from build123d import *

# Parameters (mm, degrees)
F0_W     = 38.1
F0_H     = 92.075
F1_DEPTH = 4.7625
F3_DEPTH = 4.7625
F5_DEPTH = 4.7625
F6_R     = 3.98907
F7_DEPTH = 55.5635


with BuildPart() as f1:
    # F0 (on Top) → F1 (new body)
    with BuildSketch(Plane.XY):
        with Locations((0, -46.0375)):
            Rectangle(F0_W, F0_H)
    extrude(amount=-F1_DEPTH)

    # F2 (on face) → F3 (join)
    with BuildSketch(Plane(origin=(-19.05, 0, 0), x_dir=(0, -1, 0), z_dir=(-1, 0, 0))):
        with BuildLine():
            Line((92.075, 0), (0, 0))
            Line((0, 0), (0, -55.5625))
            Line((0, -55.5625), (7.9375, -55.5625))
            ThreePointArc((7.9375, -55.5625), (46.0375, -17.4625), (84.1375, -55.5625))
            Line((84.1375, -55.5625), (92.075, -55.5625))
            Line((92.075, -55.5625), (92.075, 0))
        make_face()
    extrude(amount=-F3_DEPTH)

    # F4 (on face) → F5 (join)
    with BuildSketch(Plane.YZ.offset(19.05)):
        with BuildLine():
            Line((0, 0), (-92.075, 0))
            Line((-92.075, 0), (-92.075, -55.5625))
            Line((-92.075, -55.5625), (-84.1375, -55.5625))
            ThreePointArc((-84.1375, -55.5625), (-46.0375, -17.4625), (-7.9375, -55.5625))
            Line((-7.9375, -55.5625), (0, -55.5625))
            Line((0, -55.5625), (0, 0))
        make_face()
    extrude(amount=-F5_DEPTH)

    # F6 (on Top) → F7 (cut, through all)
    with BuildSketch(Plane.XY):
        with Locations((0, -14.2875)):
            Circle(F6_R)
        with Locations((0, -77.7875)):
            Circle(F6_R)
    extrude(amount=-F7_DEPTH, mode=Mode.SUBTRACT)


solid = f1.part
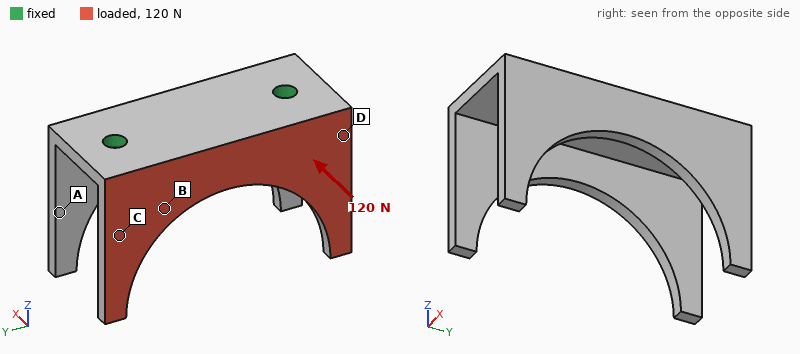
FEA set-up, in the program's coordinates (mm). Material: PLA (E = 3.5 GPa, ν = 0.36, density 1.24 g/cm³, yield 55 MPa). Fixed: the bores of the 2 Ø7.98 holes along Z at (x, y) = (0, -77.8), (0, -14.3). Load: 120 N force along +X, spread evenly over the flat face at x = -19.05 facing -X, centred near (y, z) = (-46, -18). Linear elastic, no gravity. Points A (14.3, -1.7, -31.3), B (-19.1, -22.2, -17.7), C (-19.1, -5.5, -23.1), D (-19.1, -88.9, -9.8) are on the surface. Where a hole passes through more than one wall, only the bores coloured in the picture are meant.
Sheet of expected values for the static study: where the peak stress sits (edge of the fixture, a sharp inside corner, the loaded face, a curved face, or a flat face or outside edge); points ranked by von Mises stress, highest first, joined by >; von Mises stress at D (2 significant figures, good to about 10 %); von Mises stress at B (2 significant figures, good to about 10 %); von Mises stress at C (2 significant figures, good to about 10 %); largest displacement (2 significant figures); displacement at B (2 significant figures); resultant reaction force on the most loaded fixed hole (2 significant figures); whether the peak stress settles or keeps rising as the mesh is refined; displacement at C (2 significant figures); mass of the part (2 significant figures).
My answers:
edge of the fixture
D > B > C > A
4.8 MPa
3.5 MPa
2.9 MPa
1.1 mm
0.24 mm
60 N
keeps rising
0.37 mm
48 g
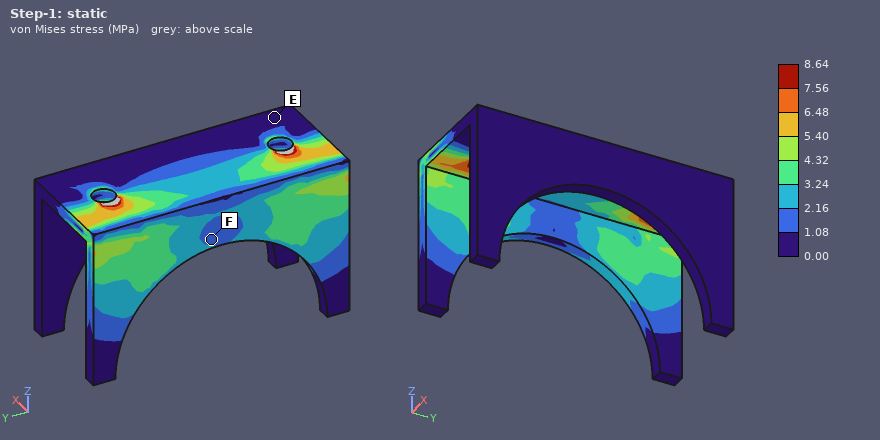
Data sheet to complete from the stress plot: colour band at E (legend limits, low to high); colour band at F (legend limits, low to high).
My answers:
0.00 to 1.08 MPa
1.08 to 2.16 MPa
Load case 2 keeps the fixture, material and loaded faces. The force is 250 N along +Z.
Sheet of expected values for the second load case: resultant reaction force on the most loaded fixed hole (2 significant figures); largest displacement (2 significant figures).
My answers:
130 N
1.0 mm
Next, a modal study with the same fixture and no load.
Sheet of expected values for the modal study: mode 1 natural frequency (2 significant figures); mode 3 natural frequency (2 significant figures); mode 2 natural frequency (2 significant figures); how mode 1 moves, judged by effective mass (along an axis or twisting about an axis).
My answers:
530 Hz
590 Hz
570 Hz
along X
